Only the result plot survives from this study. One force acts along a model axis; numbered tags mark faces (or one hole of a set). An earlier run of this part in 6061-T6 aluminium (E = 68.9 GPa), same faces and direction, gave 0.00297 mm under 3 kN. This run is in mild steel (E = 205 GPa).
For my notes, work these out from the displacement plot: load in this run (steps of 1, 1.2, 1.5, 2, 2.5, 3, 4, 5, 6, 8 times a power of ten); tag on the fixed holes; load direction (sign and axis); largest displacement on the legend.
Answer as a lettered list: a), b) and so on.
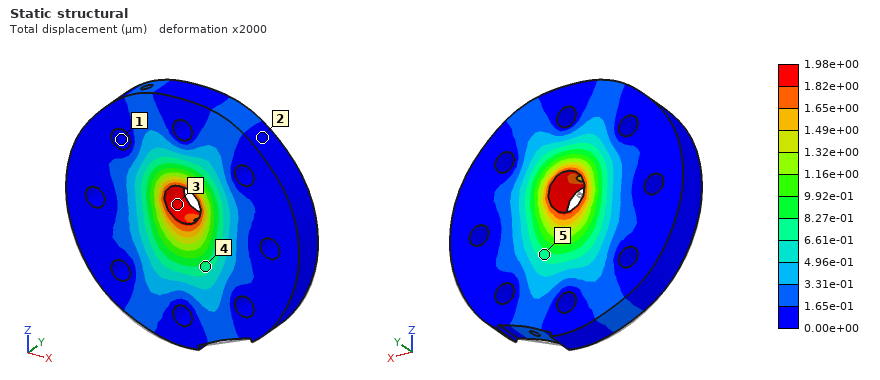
a) 6 kN
b) 1
c) +Z
d) 1.98e+00 µm
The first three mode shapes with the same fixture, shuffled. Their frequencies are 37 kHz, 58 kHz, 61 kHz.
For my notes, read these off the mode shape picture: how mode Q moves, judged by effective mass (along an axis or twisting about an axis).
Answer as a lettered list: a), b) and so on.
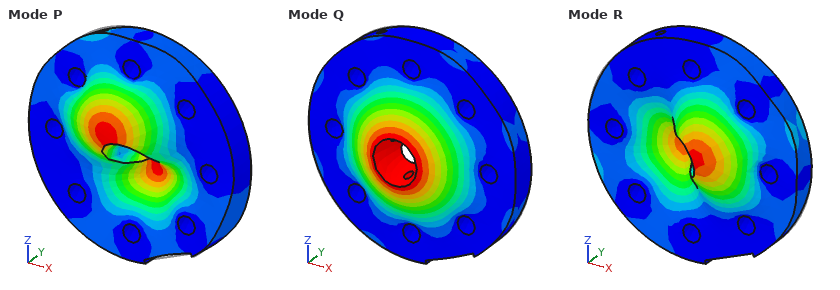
a) along Y
